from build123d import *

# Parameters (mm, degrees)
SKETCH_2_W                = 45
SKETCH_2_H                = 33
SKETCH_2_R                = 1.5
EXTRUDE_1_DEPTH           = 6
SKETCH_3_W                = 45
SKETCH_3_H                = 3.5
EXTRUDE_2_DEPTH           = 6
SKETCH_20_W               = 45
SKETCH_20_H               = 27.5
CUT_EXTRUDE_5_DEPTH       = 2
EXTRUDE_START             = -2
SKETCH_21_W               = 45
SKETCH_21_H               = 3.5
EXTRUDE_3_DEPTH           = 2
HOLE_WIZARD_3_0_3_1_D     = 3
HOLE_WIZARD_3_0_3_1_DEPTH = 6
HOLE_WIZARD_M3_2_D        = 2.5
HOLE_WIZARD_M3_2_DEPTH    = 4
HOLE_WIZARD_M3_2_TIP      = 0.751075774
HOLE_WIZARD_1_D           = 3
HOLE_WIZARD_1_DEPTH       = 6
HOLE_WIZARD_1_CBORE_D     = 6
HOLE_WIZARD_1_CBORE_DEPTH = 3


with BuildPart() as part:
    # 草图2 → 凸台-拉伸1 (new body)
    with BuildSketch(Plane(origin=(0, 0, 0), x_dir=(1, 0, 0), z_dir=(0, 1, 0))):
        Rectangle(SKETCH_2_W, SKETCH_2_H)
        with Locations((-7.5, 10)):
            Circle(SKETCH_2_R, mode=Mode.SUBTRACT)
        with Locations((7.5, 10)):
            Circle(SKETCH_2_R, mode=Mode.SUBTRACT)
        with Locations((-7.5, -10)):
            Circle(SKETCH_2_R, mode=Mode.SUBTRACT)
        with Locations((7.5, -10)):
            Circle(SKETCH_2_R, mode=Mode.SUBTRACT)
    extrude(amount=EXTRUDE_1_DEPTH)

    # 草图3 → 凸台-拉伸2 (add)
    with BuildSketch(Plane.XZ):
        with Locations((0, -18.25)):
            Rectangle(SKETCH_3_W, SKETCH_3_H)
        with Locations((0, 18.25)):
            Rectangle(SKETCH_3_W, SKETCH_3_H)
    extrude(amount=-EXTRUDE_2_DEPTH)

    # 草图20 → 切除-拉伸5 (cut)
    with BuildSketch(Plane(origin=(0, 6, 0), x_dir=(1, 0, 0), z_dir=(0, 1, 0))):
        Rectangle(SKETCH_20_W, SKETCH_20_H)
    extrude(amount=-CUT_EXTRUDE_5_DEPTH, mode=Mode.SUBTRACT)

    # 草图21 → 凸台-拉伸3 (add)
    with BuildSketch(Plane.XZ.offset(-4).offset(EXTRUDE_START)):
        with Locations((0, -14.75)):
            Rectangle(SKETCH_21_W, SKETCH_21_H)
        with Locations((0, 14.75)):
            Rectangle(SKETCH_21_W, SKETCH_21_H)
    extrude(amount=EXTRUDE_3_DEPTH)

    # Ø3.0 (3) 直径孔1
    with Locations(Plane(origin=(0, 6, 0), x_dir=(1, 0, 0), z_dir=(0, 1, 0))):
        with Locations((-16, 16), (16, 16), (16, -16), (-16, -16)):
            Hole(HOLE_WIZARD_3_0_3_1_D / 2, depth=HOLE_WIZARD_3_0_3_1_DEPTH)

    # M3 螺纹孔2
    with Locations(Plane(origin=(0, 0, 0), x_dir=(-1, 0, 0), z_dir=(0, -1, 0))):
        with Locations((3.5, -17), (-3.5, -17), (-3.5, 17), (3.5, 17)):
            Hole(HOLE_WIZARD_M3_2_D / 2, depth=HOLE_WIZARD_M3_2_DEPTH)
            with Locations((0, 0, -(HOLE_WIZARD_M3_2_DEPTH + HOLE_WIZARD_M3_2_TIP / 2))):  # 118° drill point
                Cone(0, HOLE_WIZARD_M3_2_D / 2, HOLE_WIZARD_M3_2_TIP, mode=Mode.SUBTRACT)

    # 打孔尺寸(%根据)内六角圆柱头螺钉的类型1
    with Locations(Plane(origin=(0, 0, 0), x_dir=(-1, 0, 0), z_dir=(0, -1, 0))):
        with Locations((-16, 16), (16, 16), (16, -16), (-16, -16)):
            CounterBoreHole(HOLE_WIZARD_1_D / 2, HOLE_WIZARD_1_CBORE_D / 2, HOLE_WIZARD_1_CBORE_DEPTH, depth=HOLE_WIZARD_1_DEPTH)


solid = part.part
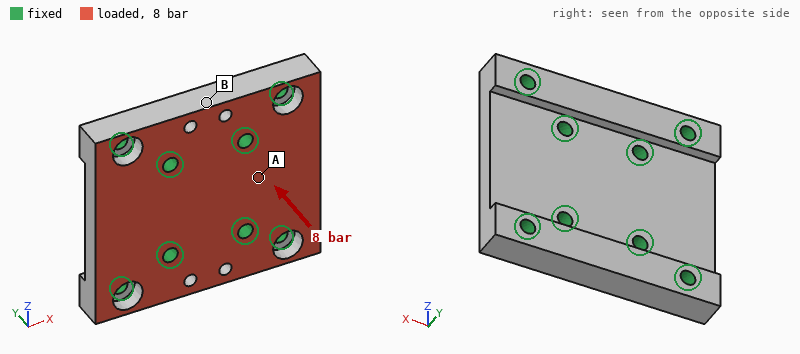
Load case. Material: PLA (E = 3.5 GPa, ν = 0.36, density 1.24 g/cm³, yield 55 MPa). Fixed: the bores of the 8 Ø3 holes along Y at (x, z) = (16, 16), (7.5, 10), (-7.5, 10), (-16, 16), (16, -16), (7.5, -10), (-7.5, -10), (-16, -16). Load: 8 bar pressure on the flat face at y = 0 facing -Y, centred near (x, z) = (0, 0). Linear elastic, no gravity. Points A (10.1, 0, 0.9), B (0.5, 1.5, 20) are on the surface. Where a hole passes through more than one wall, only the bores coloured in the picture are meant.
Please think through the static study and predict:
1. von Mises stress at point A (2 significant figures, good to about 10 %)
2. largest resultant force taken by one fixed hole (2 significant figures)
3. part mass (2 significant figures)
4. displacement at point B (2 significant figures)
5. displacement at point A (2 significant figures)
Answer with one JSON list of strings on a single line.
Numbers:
["6.7 MPa", "200 N", "9.7 g", "0.019 mm", "0.041 mm"]
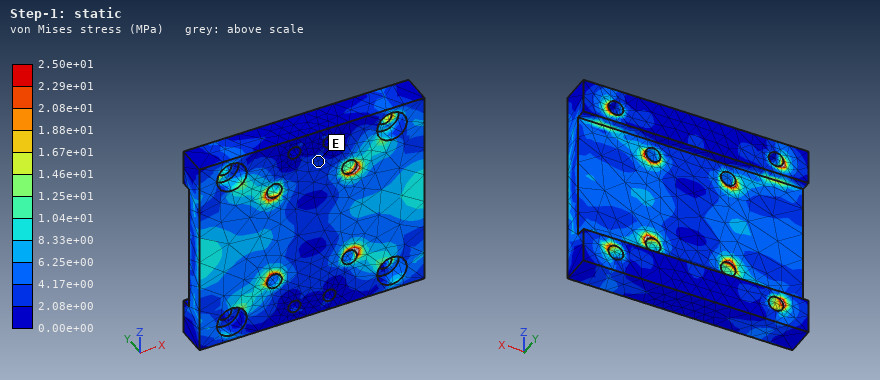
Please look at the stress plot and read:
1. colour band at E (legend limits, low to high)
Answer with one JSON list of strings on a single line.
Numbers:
["2.08e+00 to 4.17e+00 MPa"]
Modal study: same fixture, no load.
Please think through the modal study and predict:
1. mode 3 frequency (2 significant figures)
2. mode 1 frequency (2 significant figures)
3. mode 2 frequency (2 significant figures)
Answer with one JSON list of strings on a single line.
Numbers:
["11 kHz", "7500 Hz", "7500 Hz"]
